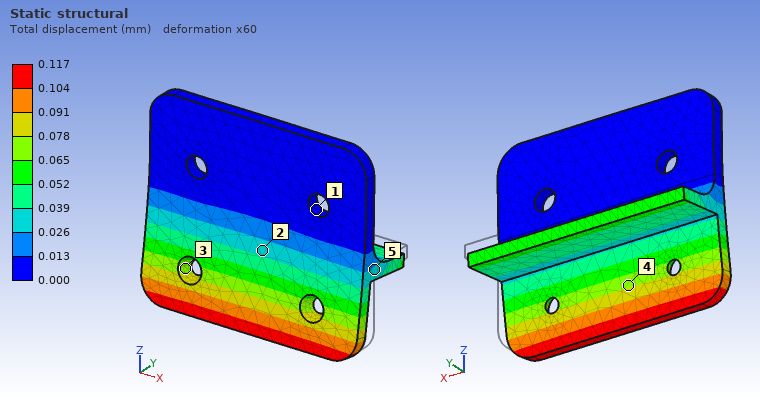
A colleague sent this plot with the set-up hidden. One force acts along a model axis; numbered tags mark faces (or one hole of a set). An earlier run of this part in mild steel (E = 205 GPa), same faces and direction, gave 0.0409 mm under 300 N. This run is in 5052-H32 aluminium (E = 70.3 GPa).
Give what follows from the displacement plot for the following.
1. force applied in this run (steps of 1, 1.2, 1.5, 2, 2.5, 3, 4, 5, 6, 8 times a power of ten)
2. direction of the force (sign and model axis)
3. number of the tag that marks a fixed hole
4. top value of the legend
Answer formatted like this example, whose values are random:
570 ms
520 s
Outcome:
300 N
-Y
1
0.117 mm
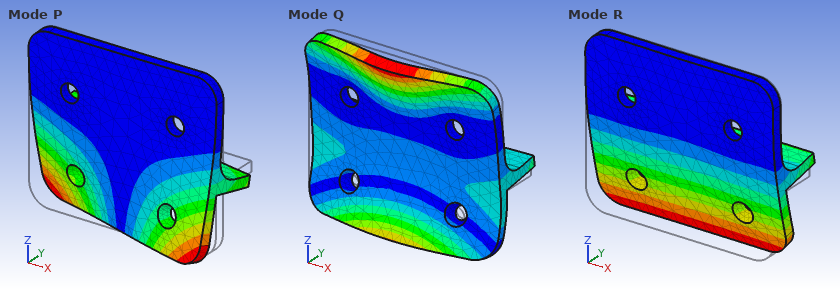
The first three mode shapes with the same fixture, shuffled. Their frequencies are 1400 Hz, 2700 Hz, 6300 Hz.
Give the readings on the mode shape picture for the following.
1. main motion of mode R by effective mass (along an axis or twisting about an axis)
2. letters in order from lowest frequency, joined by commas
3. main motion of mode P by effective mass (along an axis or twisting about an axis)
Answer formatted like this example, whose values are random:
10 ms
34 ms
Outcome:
along Y
R, P, Q
twisting about Z
